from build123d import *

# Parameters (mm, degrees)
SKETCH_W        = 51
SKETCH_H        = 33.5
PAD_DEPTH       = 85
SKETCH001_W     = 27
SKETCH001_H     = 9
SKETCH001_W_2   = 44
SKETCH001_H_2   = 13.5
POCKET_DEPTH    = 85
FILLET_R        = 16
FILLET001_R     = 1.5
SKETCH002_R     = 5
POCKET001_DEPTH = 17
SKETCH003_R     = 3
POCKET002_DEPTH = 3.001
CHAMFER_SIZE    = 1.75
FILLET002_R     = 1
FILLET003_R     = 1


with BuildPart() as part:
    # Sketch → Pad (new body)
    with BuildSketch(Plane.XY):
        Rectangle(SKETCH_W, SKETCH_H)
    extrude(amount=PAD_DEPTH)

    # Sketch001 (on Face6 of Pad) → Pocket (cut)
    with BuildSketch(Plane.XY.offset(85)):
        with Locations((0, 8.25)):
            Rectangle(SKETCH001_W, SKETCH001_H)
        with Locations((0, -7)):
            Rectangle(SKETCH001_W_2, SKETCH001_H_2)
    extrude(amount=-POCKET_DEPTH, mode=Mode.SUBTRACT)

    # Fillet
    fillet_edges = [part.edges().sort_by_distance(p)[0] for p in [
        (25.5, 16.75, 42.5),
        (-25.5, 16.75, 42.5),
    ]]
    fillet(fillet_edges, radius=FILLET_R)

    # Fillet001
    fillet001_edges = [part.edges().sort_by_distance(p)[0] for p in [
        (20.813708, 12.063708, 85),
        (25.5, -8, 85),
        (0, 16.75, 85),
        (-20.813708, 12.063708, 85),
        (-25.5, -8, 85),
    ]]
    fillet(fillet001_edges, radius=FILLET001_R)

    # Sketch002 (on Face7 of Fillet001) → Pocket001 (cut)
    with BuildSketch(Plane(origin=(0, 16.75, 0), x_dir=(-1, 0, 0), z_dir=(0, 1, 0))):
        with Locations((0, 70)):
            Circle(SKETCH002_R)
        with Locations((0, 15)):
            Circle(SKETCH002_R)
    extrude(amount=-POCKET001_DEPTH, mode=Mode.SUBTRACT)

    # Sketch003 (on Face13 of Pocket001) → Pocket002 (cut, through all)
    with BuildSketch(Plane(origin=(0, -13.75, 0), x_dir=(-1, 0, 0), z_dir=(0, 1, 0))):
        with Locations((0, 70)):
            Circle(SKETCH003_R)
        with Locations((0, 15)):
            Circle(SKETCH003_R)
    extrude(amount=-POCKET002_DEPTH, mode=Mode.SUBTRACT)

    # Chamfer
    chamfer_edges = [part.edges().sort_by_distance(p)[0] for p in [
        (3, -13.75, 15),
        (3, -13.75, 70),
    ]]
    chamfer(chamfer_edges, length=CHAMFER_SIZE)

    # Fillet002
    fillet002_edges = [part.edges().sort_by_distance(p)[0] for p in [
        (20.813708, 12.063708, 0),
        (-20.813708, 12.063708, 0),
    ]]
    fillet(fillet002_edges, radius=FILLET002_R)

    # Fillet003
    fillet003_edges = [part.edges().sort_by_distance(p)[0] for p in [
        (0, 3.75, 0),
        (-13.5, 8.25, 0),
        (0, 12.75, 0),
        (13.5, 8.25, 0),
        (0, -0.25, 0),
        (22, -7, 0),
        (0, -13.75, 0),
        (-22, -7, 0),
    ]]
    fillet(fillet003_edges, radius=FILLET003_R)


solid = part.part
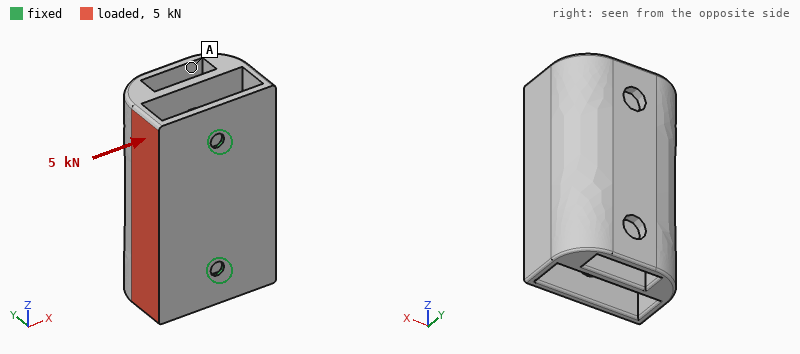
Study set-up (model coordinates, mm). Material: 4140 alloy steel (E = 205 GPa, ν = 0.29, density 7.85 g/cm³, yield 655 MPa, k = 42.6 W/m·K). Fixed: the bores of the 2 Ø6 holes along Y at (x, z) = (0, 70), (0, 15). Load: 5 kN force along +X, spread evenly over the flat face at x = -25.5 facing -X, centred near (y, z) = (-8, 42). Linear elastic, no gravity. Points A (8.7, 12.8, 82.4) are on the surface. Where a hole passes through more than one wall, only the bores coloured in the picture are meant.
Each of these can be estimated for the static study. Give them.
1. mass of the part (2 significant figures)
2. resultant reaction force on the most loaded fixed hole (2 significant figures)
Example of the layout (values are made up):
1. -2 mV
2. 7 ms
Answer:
1. 500 g
2. 2.5 kN
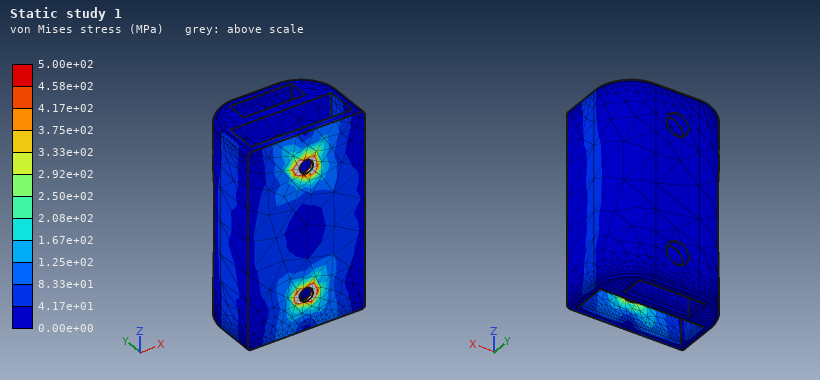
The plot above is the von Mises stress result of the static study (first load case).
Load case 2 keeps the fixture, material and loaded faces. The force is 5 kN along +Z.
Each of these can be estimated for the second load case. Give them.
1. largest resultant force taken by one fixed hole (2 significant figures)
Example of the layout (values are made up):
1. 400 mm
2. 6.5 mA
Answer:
1. 3.4 kN
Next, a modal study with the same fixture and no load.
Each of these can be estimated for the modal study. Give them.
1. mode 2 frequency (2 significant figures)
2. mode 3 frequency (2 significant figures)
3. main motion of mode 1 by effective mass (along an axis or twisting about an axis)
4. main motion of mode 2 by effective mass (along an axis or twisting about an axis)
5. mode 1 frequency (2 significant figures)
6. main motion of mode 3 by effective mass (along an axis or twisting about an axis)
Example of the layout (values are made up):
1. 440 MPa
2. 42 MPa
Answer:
1. 1400 Hz
2. 1600 Hz
3. along X
4. along Z
5. 570 Hz
6. along Y
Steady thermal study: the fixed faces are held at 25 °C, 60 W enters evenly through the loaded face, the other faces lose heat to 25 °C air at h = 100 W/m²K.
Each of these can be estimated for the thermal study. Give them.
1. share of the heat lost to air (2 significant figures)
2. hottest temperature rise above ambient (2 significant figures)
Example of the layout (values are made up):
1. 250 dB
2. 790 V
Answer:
1. 82 %
2. 49 K
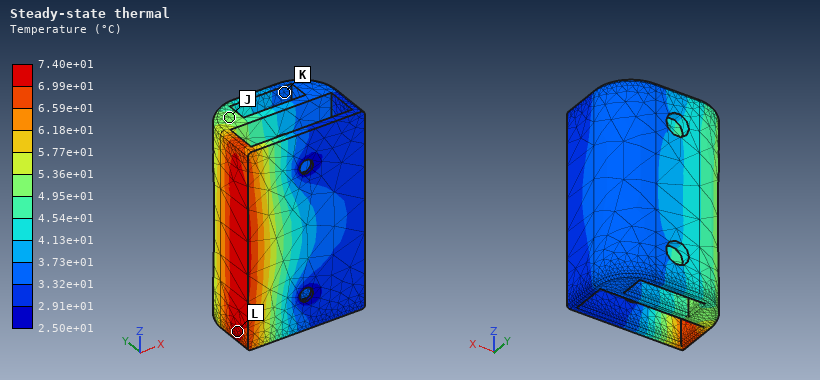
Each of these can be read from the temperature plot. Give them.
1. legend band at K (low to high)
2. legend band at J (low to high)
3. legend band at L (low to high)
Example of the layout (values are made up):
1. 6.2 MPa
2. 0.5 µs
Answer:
1. 3.32e+01 to 3.73e+01 °C
2. 4.95e+01 to 5.36e+01 °C
3. 6.99e+01 to 7.40e+01 °C
